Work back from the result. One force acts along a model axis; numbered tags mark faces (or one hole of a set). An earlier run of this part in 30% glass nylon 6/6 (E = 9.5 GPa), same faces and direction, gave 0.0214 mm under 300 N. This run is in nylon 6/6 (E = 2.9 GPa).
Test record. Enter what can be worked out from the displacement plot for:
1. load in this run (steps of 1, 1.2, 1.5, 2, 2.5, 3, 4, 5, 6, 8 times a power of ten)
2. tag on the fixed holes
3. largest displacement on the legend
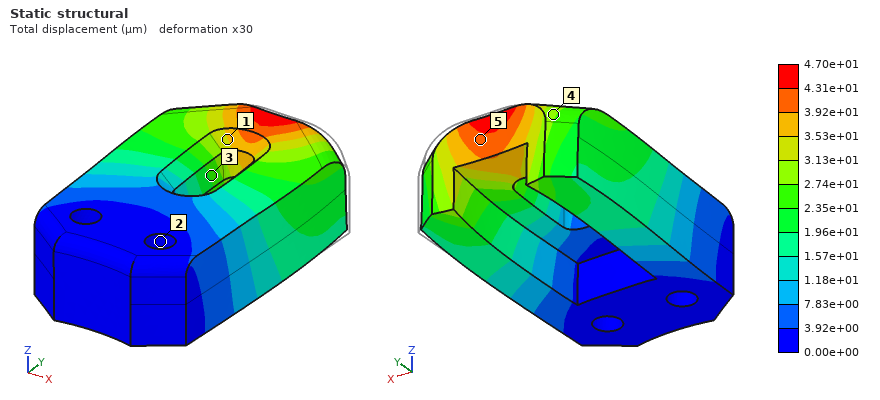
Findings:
200 N
2
4.70e+01 µm
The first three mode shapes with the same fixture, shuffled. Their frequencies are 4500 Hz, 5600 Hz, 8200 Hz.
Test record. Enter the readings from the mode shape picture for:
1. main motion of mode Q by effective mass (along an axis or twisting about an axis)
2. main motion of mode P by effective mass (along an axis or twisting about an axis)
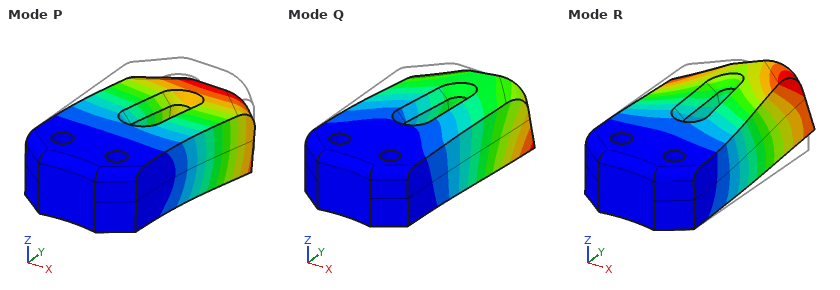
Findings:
along X
along Z
